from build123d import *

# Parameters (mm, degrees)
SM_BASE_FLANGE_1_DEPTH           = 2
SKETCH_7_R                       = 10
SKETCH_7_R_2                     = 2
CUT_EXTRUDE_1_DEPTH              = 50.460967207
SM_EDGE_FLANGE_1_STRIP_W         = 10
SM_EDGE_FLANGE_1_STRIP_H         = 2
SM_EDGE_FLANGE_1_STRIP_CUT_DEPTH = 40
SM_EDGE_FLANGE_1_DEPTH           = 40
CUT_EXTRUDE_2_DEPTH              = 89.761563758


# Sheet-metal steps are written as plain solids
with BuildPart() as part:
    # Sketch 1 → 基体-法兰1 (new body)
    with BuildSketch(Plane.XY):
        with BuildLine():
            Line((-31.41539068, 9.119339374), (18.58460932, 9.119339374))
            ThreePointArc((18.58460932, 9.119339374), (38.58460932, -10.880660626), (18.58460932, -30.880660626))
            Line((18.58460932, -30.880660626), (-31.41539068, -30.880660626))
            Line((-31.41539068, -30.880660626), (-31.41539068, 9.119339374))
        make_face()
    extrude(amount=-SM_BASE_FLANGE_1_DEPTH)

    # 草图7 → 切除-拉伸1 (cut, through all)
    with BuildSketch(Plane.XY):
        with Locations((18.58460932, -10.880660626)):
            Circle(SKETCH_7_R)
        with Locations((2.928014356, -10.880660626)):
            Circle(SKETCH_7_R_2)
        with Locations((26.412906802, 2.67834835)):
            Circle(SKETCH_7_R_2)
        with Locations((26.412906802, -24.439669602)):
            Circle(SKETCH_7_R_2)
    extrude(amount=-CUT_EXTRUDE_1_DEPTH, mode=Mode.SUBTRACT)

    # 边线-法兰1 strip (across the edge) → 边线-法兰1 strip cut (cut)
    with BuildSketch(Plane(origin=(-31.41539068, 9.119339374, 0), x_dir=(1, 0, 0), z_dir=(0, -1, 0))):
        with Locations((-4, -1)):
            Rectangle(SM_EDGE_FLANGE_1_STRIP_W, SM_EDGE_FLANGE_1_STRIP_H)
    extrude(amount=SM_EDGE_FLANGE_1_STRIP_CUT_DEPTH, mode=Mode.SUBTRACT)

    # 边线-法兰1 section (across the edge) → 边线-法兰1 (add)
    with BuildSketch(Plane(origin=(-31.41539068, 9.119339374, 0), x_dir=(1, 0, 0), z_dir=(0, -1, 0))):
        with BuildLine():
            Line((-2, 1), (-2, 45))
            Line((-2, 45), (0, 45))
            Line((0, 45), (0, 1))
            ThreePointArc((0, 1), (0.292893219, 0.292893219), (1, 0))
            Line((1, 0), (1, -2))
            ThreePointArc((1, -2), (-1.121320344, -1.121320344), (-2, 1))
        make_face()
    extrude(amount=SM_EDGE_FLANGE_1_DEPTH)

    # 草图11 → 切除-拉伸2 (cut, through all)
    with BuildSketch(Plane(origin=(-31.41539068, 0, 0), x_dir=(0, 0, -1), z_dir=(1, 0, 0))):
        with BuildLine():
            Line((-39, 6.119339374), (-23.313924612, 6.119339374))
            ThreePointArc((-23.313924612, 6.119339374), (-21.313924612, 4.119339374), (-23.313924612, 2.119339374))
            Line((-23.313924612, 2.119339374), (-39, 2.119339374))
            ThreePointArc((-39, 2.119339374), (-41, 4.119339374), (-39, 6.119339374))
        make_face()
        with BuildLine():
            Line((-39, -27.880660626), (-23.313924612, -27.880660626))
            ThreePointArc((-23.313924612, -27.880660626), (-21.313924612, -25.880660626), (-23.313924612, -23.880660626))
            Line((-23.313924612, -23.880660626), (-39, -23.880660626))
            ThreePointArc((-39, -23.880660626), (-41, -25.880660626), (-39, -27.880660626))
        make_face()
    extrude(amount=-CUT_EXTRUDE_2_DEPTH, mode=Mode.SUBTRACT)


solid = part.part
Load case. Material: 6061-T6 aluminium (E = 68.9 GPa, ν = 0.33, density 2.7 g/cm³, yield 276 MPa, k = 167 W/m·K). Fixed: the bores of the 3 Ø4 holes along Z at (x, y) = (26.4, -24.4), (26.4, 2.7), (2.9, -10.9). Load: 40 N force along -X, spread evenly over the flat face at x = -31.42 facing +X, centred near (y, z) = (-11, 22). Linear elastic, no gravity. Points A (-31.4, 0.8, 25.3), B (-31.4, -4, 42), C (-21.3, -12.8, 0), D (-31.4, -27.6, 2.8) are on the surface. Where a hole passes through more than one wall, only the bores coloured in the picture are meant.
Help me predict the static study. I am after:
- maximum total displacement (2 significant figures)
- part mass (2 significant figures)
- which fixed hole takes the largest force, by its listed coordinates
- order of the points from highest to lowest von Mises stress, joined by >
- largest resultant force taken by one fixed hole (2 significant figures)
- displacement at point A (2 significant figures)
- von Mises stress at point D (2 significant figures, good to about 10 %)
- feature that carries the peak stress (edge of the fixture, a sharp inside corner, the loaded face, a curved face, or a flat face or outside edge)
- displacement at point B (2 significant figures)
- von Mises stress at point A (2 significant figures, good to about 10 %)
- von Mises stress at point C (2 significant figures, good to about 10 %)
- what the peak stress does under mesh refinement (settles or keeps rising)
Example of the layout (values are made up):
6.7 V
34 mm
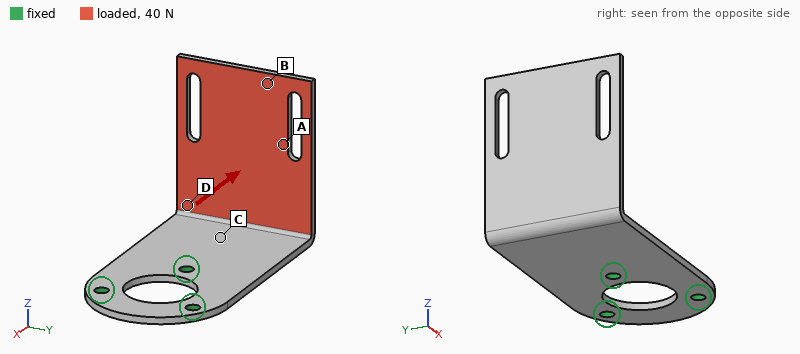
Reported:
1.1 mm
21 g
(2.9, -10.9)
C > D > A > B
33 N
0.62 mm
24 MPa
edge of the fixture
1.00 mm
8.1 MPa
32 MPa
keeps rising
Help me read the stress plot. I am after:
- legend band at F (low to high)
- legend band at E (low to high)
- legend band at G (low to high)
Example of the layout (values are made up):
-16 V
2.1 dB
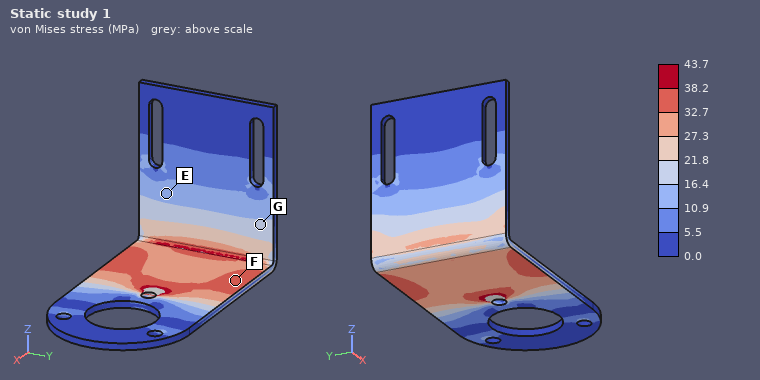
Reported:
32.7 to 38.2 MPa
10.9 to 16.4 MPa
16.4 to 21.8 MPa
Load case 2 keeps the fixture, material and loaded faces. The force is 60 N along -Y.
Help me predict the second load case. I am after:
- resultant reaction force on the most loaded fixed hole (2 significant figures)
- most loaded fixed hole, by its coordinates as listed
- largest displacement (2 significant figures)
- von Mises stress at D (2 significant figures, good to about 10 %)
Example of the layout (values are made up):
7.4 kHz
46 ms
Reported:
78 N
(2.9, -10.9)
0.85 mm
30 MPa
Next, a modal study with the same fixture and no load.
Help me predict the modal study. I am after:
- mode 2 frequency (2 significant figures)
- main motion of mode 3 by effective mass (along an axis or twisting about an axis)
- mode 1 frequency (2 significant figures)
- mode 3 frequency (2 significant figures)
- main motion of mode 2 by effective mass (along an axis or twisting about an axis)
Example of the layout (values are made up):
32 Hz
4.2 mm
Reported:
520 Hz
along Z
350 Hz
950 Hz
along Y
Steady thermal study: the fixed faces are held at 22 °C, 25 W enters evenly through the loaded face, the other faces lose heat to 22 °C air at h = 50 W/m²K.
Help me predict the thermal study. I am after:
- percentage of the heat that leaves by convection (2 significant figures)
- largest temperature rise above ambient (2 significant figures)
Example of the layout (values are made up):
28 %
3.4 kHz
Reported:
45 %
77 K
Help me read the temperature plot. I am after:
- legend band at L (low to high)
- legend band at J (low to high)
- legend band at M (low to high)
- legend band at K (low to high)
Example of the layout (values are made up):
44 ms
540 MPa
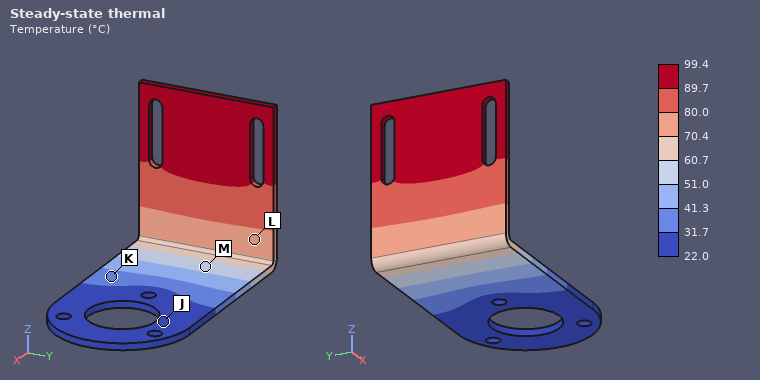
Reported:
70.4 to 80.0 °C
22.0 to 31.7 °C
51.0 to 60.7 °C
31.7 to 41.3 °C
